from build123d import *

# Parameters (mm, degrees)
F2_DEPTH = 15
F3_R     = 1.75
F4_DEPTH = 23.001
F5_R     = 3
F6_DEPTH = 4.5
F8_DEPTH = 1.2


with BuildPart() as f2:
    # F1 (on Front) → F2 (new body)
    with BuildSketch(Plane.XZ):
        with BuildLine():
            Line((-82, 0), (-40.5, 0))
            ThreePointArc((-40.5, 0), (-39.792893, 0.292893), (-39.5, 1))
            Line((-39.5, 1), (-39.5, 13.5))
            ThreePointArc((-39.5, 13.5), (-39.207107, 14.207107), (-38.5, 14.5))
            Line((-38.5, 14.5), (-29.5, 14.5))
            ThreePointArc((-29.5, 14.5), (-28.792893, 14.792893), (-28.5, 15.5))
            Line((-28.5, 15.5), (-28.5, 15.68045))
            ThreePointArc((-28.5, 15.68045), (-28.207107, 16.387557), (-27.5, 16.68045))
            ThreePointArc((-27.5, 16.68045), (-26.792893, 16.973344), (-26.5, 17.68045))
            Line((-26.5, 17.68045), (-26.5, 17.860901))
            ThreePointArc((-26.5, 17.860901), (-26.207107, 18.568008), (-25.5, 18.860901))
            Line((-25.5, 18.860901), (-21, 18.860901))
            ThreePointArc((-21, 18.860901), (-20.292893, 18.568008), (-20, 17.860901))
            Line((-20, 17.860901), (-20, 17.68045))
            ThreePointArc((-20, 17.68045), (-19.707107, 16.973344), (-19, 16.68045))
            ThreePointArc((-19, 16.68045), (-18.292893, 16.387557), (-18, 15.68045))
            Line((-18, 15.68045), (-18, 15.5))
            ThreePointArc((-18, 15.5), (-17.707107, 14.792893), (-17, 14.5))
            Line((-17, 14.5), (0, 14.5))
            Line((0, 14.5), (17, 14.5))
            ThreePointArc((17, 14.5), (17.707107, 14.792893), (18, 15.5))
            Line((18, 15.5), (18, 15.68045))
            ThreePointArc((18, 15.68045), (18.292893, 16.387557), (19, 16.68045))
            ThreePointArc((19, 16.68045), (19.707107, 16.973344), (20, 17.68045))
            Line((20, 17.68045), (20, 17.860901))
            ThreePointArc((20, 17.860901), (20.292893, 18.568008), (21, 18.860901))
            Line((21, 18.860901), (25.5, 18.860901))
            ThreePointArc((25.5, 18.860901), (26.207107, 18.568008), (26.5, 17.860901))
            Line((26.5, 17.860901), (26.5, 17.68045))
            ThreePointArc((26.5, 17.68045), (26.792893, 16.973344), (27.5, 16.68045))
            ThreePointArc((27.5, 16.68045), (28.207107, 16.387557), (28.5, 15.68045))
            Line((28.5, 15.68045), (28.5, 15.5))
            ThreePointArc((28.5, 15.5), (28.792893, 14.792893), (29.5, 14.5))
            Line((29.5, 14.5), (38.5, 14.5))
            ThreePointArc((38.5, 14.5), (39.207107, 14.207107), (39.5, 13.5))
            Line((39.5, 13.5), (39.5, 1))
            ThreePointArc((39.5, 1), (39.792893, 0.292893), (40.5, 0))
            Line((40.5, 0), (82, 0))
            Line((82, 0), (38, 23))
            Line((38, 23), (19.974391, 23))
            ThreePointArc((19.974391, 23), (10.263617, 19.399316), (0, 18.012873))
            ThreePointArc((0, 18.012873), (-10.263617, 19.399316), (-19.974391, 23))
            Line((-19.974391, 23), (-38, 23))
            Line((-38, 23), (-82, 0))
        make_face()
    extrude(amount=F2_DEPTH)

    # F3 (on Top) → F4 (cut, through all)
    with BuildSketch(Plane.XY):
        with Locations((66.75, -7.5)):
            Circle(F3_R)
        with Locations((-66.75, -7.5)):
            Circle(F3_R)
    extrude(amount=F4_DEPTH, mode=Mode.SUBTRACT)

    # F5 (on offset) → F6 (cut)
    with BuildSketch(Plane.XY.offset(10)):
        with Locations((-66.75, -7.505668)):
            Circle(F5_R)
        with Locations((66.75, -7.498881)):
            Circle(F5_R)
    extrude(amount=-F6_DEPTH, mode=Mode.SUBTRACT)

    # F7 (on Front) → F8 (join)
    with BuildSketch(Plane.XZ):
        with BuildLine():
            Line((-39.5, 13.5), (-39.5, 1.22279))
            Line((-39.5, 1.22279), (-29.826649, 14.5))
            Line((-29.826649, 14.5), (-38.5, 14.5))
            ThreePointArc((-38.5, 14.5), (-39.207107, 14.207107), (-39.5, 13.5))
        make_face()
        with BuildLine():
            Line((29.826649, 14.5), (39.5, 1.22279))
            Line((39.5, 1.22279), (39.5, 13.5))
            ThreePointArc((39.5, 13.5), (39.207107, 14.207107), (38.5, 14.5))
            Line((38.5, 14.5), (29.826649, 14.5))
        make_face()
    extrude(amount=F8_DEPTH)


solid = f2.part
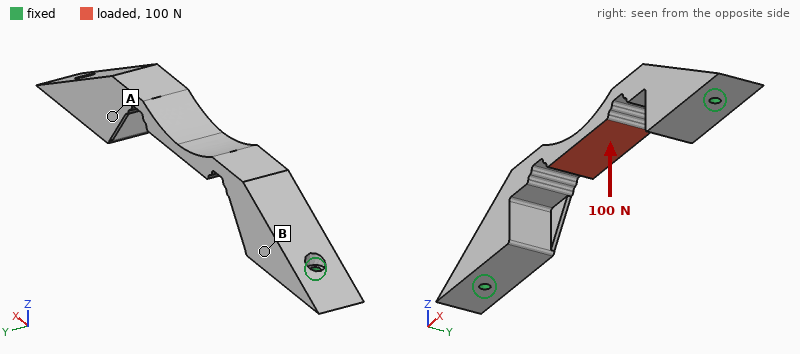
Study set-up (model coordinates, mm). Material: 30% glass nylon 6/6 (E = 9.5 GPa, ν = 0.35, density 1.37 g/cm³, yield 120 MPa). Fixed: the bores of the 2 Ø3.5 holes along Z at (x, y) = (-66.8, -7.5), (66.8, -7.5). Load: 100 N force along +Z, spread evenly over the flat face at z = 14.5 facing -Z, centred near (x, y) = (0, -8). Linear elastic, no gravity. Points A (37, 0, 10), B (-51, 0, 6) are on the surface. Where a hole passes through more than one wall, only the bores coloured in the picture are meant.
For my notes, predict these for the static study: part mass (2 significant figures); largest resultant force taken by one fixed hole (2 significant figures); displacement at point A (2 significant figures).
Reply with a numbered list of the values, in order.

1. 29 g
2. 98 N
3. 0.066 mm
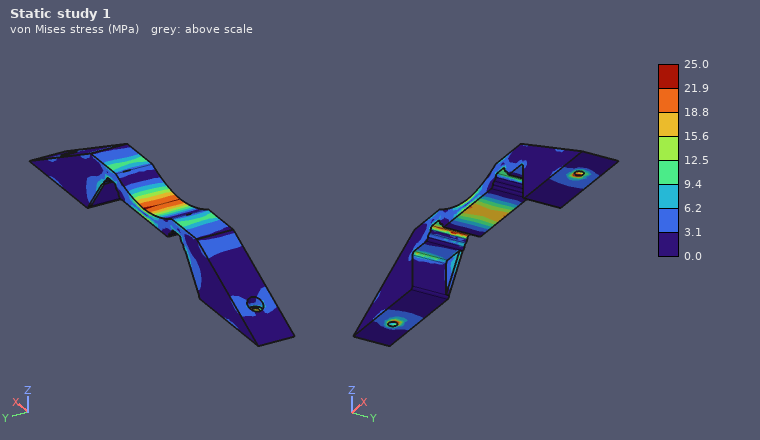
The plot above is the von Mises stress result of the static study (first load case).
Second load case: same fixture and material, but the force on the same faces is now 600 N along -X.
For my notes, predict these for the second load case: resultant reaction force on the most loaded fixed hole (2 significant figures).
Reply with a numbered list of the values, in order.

1. 300 N
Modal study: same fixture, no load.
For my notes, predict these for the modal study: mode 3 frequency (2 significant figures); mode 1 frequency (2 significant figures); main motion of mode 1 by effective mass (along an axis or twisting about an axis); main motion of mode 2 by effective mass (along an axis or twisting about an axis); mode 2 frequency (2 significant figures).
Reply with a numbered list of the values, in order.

1. 1700 Hz
2. 1300 Hz
3. along Y
4. along Z
5. 1400 Hz
